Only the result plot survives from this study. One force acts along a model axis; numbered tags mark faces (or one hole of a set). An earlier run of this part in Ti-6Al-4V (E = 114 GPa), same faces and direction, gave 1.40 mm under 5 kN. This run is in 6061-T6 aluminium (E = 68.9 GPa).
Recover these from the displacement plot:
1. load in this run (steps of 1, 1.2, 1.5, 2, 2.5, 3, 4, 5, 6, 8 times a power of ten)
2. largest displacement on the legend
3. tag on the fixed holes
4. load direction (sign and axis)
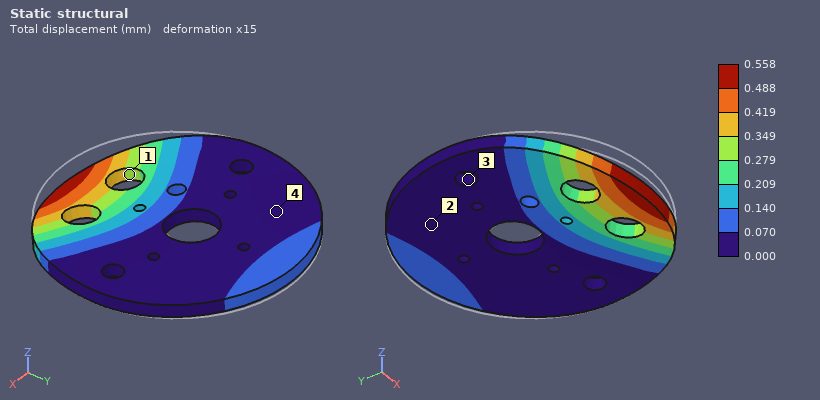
1.2 kN
0.558 mm
3
-Z
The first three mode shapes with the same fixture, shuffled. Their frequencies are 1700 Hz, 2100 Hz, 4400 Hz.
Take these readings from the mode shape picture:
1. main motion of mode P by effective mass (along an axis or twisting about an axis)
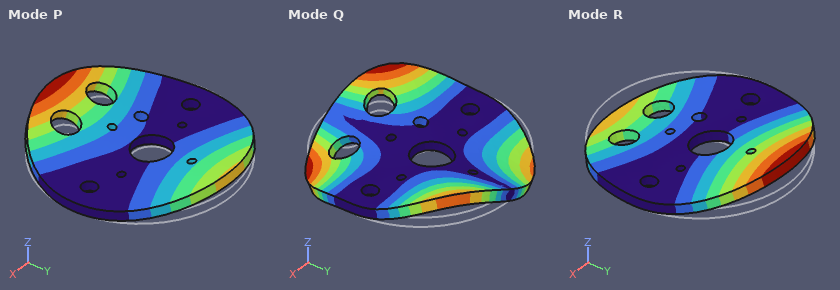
along Z
